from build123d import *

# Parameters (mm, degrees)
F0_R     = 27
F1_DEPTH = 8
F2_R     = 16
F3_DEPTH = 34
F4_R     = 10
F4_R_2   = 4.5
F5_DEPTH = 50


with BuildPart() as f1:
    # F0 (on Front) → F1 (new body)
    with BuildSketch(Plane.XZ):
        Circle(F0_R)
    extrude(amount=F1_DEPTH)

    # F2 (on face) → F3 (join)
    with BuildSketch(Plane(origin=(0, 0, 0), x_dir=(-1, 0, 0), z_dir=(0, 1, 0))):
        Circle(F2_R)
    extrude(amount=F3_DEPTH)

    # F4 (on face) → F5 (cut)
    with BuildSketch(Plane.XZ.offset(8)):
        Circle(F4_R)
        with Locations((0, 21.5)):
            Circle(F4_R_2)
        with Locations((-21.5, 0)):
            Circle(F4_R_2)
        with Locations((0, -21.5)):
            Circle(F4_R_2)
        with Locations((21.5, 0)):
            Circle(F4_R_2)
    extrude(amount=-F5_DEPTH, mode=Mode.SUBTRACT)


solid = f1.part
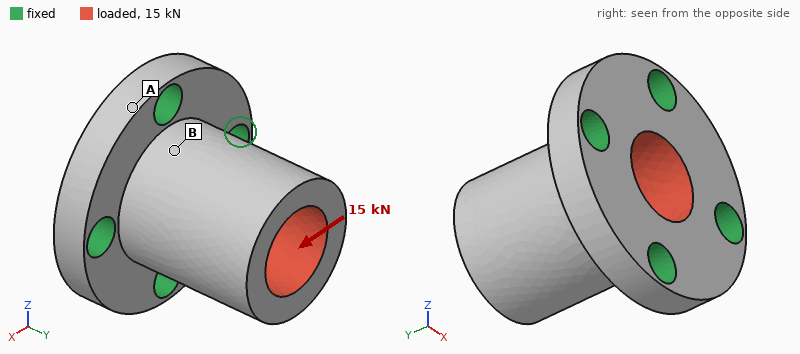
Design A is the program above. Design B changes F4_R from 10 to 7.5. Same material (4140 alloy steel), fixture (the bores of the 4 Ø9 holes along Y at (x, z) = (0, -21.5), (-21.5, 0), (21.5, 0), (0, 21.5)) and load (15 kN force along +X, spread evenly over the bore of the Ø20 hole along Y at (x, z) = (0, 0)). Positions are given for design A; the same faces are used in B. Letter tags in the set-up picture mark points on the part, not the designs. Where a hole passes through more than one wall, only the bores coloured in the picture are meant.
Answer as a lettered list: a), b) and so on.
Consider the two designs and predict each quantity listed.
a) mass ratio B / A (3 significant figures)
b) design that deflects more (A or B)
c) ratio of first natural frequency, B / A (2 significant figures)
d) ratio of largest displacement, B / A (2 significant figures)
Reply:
a) 1.19
b) A
c) 0.96
d) 0.85
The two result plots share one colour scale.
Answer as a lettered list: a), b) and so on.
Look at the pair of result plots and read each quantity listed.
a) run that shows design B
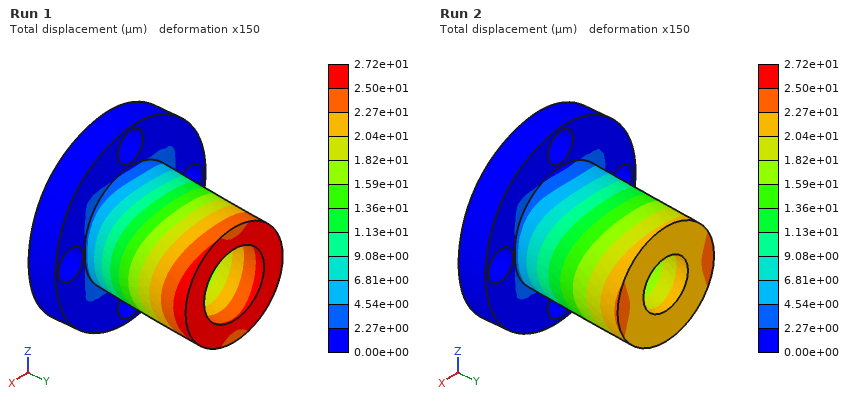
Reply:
a) Run 2
